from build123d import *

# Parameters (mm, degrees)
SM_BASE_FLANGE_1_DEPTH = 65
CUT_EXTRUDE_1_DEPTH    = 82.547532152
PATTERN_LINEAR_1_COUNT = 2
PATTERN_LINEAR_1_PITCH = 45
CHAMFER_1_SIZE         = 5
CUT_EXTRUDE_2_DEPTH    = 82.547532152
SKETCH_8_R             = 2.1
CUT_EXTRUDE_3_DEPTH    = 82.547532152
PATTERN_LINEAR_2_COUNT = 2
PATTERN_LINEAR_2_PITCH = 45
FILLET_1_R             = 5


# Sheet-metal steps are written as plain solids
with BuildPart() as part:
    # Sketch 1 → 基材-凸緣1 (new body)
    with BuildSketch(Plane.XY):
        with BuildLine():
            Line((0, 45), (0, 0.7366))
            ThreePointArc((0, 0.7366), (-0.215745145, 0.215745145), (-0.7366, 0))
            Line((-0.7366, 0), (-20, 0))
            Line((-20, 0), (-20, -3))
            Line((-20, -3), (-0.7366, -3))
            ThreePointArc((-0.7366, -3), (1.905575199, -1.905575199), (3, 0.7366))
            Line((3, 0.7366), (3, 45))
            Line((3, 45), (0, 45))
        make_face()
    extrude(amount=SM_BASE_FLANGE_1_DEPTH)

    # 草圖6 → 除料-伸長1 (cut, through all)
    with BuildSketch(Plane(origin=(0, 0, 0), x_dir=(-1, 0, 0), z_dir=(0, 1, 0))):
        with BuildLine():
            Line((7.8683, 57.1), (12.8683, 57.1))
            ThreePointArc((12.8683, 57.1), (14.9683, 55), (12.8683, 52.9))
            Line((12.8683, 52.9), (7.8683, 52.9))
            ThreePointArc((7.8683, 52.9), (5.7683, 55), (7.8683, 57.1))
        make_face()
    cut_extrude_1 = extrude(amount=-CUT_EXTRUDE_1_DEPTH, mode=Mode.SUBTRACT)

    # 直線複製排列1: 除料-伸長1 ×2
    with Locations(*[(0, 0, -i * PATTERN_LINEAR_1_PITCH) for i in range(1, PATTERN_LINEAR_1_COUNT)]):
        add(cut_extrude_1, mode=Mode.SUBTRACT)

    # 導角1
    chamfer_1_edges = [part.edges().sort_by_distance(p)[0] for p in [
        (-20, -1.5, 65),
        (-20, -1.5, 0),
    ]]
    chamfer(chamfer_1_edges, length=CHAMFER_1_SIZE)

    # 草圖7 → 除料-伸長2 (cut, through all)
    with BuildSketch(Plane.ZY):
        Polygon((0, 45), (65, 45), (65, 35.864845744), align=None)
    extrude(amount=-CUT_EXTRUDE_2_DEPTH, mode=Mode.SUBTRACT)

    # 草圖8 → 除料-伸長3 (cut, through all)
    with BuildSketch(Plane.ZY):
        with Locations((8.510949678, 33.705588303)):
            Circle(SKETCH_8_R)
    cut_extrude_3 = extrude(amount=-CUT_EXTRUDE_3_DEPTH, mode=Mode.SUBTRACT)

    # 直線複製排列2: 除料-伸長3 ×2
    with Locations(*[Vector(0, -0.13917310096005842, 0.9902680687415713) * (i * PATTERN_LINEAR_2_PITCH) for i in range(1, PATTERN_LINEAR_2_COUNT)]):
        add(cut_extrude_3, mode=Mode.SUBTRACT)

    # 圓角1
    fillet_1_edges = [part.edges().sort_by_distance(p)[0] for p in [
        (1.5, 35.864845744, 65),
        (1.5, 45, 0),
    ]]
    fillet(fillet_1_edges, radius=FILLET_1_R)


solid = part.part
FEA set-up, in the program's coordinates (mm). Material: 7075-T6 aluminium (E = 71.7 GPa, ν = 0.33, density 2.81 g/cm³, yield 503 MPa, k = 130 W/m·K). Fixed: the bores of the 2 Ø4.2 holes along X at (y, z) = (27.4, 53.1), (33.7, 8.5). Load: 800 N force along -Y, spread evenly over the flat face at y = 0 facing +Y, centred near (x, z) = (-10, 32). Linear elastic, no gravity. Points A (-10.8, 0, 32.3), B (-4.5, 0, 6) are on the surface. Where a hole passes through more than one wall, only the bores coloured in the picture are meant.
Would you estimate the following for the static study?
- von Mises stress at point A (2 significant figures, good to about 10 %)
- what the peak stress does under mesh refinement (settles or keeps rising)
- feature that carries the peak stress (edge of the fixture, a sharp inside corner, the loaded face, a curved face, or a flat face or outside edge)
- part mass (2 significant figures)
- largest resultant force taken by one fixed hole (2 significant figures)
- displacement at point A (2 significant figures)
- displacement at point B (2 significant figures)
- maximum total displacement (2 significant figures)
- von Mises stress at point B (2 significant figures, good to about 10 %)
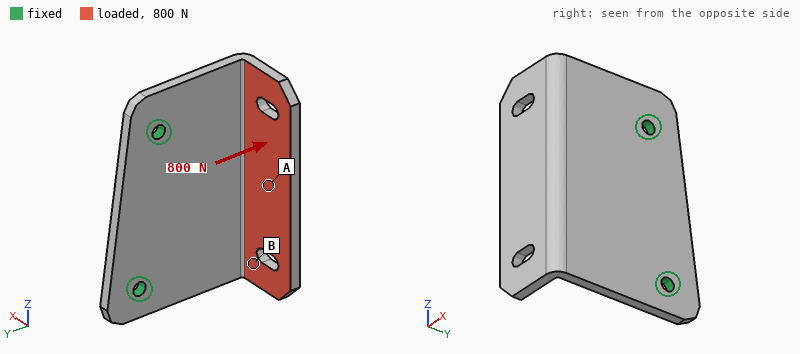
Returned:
19 MPa
keeps rising
edge of the fixture
33 g
430 N
0.57 mm
0.51 mm
0.90 mm
46 MPa
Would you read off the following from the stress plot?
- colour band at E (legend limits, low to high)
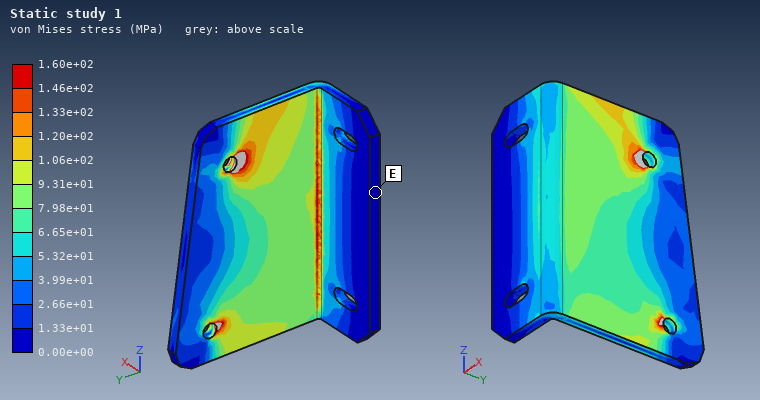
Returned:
0.00e+00 to 1.33e+01 MPa
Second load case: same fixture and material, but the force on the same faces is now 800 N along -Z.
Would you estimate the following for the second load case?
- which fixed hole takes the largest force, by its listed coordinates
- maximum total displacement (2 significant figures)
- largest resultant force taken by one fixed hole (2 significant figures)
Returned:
(27.4, 53.1)
0.41 mm
730 N
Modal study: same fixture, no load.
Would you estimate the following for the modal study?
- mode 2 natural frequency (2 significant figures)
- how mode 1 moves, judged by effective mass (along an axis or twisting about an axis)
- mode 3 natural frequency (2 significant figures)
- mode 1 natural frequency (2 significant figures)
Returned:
2000 Hz
along X
3700 Hz
1100 Hz
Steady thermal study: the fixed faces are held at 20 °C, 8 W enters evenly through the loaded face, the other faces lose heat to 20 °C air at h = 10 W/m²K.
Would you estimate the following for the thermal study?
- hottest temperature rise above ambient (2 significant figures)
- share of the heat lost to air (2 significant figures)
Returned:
15 K
6.8 %
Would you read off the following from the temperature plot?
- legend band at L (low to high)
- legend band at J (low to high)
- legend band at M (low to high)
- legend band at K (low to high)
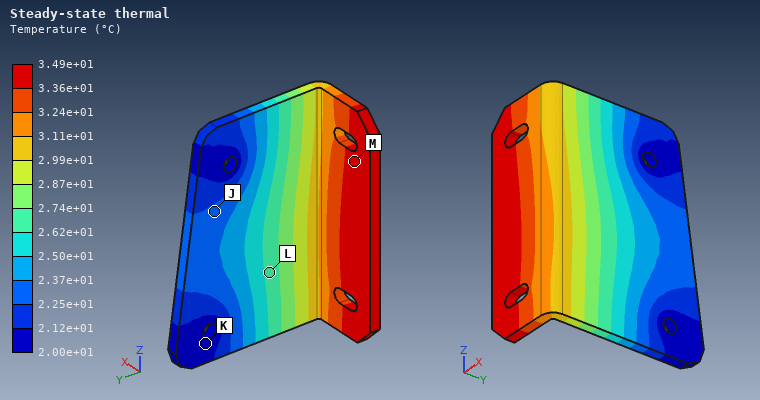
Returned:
2.62e+01 to 2.74e+01 °C
2.25e+01 to 2.37e+01 °C
3.36e+01 to 3.49e+01 °C
2.00e+01 to 2.12e+01 °C
